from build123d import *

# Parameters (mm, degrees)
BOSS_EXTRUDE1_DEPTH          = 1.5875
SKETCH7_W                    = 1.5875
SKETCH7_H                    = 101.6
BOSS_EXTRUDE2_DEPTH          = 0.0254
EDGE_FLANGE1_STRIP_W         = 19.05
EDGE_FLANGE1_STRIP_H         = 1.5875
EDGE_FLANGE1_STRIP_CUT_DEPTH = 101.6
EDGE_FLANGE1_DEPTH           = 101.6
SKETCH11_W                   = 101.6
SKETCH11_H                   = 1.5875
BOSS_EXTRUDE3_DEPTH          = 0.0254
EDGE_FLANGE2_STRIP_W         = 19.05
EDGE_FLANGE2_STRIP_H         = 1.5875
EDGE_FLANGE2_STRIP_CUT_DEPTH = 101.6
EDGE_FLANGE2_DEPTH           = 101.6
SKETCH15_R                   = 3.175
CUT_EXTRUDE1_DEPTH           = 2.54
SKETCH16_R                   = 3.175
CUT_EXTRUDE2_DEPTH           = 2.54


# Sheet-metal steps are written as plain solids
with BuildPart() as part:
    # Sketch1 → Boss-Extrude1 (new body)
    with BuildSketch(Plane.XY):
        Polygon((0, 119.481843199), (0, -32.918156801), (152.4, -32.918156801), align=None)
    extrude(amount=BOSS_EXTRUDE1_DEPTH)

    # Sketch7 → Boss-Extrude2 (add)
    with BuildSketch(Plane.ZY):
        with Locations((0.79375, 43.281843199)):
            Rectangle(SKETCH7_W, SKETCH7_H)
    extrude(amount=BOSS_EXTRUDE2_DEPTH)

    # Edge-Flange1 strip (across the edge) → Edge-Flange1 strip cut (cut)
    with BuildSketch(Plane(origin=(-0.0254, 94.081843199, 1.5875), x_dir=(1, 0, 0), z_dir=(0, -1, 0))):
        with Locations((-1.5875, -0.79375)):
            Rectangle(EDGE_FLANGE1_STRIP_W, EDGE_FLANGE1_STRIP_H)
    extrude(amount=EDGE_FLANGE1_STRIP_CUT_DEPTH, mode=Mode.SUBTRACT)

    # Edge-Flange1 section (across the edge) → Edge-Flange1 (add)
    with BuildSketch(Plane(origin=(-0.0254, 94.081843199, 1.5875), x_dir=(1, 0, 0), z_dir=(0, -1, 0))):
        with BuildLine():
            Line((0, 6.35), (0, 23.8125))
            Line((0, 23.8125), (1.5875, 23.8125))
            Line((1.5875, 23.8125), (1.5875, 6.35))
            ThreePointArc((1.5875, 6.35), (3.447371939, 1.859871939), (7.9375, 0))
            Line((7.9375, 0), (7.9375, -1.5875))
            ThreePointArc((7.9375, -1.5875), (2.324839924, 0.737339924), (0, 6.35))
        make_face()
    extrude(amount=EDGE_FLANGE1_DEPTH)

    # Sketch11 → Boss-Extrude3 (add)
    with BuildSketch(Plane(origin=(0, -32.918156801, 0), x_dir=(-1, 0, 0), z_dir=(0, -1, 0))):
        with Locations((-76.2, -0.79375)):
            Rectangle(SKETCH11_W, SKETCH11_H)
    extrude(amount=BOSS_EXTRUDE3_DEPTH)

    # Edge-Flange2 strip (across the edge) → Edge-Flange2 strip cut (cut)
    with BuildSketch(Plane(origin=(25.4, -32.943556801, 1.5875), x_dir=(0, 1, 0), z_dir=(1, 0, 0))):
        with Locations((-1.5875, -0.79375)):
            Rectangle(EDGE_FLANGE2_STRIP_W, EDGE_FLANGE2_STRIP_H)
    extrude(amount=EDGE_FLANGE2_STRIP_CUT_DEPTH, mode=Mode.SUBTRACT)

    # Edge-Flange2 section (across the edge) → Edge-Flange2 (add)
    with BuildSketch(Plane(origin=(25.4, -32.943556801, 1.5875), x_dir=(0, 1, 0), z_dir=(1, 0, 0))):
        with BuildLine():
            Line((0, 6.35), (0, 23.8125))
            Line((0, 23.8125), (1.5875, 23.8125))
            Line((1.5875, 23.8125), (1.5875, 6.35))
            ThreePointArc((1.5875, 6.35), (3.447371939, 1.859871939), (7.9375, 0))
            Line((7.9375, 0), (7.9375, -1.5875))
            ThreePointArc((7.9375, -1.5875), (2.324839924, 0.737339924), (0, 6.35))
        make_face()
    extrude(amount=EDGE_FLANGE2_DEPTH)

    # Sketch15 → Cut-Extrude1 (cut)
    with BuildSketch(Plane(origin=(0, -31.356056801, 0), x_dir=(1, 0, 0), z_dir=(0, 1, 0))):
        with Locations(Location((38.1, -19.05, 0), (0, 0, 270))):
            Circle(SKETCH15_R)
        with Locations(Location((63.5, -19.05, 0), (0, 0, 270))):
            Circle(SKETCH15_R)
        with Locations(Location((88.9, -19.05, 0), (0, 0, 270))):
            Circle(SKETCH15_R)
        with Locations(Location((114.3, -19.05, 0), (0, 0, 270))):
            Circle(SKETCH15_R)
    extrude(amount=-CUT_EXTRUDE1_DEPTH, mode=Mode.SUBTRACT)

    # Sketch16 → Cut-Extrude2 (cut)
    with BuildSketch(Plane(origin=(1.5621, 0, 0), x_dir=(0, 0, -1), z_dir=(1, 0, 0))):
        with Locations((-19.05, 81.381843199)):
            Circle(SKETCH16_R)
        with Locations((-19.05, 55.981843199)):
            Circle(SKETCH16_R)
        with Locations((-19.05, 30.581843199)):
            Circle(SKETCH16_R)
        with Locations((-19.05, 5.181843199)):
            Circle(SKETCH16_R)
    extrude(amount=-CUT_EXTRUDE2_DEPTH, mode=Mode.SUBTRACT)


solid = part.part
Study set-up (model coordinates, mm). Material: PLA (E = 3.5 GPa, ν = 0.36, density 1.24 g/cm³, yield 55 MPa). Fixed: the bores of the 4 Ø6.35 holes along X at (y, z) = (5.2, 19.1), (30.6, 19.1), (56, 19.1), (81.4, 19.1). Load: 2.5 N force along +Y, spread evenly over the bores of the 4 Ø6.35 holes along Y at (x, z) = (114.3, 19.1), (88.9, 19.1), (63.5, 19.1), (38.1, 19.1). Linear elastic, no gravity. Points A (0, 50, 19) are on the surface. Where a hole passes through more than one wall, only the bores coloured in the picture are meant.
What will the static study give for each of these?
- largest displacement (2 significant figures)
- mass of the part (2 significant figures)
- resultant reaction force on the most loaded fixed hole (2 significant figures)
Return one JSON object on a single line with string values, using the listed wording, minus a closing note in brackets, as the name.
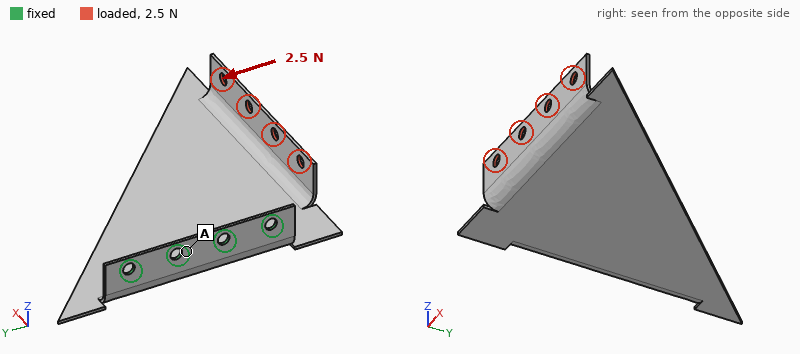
{"largest displacement": "2.3 mm", "mass of the part": "31 g", "resultant reaction force on the most loaded fixed hole": "2.6 N"}
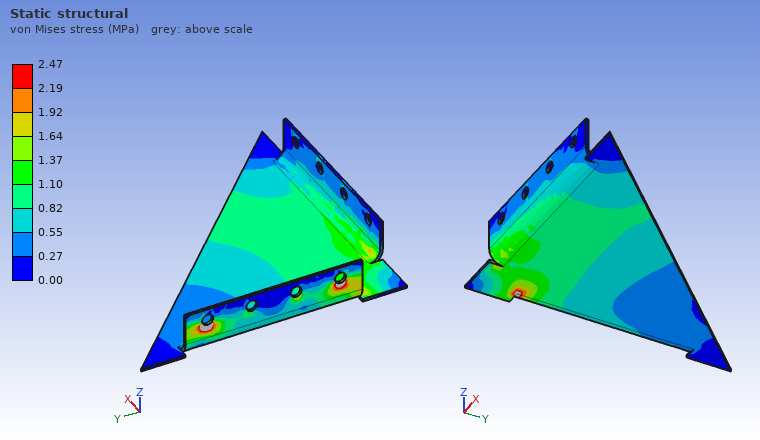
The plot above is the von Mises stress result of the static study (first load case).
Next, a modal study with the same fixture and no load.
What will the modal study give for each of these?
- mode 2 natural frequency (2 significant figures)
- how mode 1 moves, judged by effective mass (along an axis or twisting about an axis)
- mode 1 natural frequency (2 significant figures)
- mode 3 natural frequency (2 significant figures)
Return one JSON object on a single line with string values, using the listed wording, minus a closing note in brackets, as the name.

{"mode 2 natural frequency": "95 Hz", "how mode 1 moves, judged by effective mass": "along Z", "mode 1 natural frequency": "23 Hz", "mode 3 natural frequency": "130 Hz"}
